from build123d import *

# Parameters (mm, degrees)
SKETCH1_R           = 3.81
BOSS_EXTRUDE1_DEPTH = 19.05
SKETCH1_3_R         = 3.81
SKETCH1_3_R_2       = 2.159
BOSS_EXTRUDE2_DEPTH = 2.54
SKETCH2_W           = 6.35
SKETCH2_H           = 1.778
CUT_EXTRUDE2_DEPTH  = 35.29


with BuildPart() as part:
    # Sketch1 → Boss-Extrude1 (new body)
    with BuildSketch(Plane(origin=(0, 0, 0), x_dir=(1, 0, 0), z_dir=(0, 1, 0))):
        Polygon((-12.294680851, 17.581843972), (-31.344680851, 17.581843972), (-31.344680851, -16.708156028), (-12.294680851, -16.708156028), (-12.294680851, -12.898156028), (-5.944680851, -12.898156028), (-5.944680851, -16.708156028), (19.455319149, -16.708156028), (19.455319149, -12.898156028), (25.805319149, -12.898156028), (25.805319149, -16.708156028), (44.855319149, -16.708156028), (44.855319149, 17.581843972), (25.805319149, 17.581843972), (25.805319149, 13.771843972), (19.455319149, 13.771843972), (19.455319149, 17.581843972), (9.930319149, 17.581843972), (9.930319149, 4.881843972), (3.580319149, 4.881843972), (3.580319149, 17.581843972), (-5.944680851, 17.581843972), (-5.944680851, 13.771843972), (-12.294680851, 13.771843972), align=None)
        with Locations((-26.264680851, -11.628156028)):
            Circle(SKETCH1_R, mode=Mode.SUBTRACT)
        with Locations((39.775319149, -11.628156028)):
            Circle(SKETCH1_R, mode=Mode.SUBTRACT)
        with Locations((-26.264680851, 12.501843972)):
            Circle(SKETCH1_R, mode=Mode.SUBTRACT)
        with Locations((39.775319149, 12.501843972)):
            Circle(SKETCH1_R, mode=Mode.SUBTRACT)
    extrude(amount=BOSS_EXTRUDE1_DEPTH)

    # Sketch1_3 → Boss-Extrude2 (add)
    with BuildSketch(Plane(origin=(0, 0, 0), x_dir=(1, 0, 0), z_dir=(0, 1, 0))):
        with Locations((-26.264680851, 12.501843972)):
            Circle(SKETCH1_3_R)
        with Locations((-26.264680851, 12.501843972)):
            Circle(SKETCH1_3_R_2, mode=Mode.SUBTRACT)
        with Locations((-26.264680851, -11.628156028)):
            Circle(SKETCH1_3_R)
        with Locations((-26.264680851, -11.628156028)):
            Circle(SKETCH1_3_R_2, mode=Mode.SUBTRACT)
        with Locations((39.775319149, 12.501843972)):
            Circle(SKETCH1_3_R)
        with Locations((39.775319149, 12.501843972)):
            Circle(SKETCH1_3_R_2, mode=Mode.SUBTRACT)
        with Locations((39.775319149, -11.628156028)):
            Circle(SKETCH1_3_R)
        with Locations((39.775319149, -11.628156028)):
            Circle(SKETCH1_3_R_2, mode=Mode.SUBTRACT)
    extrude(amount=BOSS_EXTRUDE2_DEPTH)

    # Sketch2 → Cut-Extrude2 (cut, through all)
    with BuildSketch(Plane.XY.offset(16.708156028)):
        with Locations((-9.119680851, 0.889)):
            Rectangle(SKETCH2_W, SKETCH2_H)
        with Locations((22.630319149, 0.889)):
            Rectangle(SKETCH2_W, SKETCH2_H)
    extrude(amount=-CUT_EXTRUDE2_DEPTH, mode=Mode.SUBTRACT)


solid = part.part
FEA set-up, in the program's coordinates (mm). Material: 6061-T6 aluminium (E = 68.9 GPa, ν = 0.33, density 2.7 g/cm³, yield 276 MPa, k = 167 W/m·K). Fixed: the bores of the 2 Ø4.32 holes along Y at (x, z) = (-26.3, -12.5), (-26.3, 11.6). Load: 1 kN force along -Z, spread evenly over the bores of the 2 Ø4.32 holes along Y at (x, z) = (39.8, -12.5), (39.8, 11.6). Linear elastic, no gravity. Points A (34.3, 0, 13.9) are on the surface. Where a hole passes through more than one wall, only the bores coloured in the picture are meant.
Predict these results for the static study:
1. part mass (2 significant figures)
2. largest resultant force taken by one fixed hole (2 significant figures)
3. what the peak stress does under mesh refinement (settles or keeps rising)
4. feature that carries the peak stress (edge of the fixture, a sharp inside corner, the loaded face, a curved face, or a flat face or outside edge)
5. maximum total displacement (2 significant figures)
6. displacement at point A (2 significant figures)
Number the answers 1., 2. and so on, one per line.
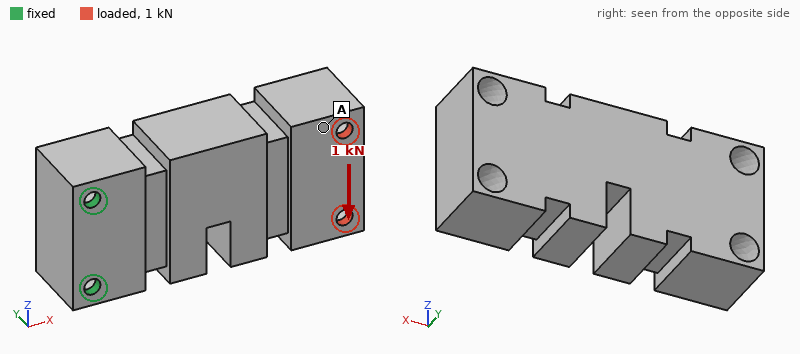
1. 120 g
2. 2.6 kN
3. keeps rising
4. edge of the fixture
5. 0.13 mm
6. 0.10 mm
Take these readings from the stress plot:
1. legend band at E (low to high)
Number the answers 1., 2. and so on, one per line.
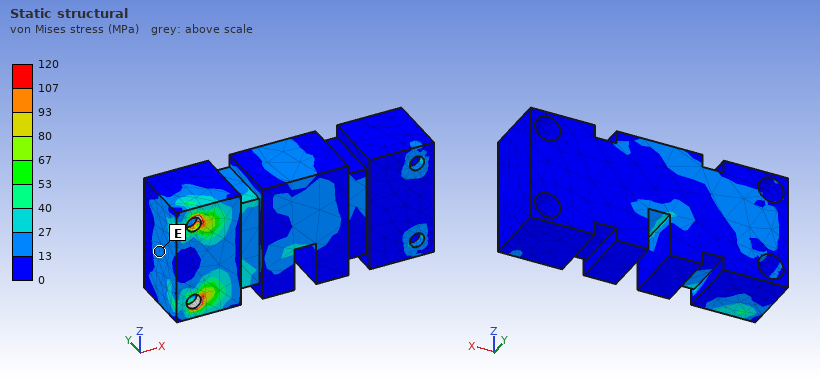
1. 13 to 27 MPa
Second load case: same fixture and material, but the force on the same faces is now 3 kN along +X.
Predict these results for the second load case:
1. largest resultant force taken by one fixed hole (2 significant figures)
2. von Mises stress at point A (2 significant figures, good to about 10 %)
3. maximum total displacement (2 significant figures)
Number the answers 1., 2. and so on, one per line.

1. 1.5 kN
2. 37 MPa
3. 78 µm
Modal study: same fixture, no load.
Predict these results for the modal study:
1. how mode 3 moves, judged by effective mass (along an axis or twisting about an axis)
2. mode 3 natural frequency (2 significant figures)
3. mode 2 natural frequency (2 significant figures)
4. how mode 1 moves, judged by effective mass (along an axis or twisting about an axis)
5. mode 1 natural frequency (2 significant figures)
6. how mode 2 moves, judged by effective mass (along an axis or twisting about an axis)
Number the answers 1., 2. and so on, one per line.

1. twisting about X
2. 6500 Hz
3. 2600 Hz
4. along Y
5. 710 Hz
6. along Z
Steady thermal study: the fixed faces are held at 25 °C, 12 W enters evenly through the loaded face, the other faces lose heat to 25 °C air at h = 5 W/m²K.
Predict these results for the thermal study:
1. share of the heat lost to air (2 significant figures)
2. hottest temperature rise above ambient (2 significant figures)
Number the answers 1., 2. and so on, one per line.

1. 3.8 %
2. 17 K
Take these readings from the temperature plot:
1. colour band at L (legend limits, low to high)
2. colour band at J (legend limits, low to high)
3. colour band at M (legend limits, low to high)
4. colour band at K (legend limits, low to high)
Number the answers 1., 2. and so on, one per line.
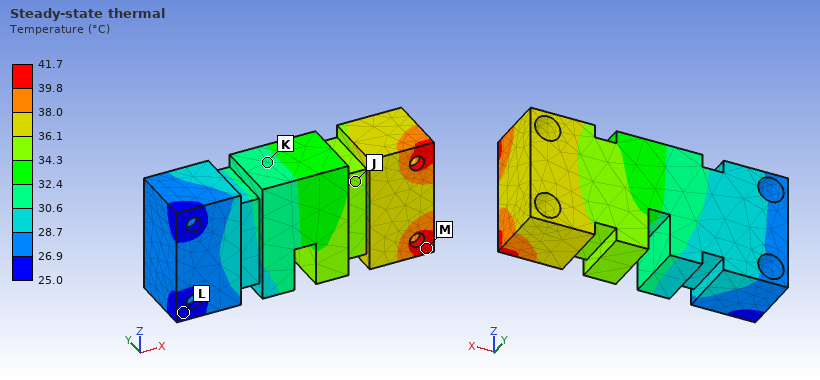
1. 25.0 to 26.9 °C
2. 34.3 to 36.1 °C
3. 39.8 to 41.7 °C
4. 30.6 to 32.4 °C
